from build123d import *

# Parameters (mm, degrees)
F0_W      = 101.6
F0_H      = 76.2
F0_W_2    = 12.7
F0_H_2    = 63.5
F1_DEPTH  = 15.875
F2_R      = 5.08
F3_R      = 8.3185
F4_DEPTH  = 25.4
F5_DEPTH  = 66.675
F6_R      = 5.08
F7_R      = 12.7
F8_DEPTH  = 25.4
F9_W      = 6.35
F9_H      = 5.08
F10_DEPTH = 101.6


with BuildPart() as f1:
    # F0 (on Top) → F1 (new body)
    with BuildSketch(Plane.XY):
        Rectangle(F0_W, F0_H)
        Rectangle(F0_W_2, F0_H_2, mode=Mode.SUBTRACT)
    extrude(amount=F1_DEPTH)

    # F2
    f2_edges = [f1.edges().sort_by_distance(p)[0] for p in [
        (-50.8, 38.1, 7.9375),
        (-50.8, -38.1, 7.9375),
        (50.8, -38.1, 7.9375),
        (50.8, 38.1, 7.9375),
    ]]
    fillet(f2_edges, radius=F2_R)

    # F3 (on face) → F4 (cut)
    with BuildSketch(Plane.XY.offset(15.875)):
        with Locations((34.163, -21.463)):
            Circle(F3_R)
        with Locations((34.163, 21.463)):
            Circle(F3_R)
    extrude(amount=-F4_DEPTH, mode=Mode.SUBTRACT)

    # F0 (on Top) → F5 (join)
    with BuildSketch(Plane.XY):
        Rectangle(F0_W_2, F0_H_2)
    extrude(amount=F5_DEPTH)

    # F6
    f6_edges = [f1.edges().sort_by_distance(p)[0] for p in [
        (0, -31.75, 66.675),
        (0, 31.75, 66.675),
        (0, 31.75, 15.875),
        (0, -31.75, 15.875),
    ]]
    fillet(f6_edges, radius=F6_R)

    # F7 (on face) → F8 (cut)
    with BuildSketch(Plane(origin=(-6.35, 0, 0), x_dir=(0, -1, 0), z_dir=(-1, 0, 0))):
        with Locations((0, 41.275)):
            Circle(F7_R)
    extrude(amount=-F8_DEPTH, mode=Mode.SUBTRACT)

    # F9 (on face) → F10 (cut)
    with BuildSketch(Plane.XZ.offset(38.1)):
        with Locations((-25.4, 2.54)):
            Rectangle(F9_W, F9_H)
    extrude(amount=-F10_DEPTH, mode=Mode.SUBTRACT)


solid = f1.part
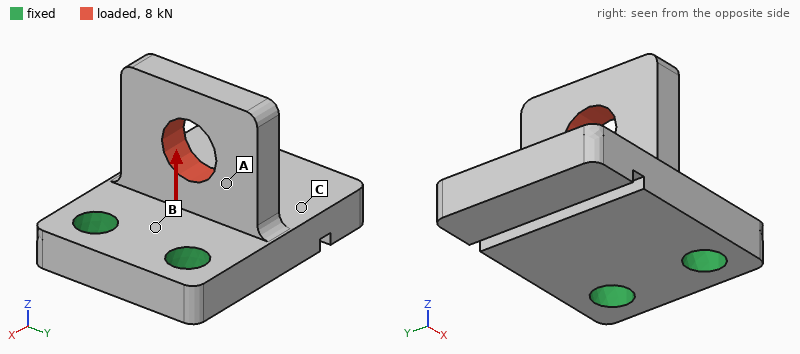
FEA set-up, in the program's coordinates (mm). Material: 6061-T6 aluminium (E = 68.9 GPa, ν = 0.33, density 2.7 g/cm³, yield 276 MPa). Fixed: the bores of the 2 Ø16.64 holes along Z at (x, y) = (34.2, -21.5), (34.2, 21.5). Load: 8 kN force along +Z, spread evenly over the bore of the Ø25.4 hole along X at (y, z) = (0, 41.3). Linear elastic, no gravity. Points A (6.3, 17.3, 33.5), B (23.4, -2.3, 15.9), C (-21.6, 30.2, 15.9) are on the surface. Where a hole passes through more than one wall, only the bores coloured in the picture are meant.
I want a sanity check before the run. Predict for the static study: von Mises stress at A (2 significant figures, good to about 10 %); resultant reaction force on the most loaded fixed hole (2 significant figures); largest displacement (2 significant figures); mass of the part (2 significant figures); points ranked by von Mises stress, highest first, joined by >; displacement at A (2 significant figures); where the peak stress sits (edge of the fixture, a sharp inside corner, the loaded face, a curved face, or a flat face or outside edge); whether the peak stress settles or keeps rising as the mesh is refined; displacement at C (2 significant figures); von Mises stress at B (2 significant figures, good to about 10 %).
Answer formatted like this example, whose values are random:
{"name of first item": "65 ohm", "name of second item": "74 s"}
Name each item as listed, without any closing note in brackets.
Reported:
{"von Mises stress at A": "15 MPa", "resultant reaction force on the most loaded fixed hole": "4.0 kN", "largest displacement": "0.15 mm", "mass of the part": "400 g", "points ranked by von Mises stress, highest first, joined by >": "B > A > C", "displacement at A": "0.063 mm", "where the peak stress sits": "edge of the fixture", "whether the peak stress settles or keeps rising as the mesh is refined": "keeps rising", "displacement at C": "0.090 mm", "von Mises stress at B": "33 MPa"}
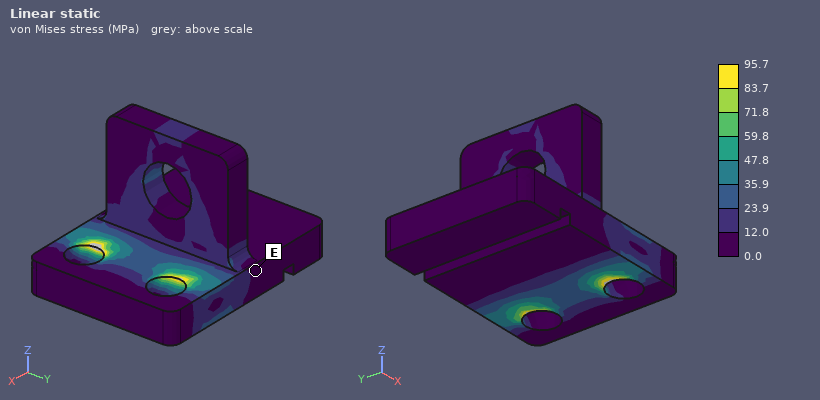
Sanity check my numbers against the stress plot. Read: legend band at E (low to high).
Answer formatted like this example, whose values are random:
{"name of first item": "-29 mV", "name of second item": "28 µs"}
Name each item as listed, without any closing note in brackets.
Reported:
{"legend band at E": "0.0 to 12.0 MPa"}
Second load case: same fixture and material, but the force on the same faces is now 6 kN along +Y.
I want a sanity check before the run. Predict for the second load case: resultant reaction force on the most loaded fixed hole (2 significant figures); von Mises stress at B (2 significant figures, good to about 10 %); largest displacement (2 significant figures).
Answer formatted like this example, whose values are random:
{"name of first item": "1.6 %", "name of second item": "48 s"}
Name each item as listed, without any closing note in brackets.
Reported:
{"resultant reaction force on the most loaded fixed hole": "5.7 kN", "von Mises stress at B": "23 MPa", "largest displacement": "91 µm"}
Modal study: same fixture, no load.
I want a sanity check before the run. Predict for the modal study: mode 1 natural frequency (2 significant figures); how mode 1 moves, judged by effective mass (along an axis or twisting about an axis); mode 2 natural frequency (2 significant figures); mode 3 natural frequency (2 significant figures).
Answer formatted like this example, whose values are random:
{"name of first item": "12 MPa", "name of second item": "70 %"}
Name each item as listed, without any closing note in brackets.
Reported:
{"mode 1 natural frequency": "1700 Hz", "how mode 1 moves, judged by effective mass": "along Z", "mode 2 natural frequency": "3600 Hz", "mode 3 natural frequency": "3700 Hz"}
